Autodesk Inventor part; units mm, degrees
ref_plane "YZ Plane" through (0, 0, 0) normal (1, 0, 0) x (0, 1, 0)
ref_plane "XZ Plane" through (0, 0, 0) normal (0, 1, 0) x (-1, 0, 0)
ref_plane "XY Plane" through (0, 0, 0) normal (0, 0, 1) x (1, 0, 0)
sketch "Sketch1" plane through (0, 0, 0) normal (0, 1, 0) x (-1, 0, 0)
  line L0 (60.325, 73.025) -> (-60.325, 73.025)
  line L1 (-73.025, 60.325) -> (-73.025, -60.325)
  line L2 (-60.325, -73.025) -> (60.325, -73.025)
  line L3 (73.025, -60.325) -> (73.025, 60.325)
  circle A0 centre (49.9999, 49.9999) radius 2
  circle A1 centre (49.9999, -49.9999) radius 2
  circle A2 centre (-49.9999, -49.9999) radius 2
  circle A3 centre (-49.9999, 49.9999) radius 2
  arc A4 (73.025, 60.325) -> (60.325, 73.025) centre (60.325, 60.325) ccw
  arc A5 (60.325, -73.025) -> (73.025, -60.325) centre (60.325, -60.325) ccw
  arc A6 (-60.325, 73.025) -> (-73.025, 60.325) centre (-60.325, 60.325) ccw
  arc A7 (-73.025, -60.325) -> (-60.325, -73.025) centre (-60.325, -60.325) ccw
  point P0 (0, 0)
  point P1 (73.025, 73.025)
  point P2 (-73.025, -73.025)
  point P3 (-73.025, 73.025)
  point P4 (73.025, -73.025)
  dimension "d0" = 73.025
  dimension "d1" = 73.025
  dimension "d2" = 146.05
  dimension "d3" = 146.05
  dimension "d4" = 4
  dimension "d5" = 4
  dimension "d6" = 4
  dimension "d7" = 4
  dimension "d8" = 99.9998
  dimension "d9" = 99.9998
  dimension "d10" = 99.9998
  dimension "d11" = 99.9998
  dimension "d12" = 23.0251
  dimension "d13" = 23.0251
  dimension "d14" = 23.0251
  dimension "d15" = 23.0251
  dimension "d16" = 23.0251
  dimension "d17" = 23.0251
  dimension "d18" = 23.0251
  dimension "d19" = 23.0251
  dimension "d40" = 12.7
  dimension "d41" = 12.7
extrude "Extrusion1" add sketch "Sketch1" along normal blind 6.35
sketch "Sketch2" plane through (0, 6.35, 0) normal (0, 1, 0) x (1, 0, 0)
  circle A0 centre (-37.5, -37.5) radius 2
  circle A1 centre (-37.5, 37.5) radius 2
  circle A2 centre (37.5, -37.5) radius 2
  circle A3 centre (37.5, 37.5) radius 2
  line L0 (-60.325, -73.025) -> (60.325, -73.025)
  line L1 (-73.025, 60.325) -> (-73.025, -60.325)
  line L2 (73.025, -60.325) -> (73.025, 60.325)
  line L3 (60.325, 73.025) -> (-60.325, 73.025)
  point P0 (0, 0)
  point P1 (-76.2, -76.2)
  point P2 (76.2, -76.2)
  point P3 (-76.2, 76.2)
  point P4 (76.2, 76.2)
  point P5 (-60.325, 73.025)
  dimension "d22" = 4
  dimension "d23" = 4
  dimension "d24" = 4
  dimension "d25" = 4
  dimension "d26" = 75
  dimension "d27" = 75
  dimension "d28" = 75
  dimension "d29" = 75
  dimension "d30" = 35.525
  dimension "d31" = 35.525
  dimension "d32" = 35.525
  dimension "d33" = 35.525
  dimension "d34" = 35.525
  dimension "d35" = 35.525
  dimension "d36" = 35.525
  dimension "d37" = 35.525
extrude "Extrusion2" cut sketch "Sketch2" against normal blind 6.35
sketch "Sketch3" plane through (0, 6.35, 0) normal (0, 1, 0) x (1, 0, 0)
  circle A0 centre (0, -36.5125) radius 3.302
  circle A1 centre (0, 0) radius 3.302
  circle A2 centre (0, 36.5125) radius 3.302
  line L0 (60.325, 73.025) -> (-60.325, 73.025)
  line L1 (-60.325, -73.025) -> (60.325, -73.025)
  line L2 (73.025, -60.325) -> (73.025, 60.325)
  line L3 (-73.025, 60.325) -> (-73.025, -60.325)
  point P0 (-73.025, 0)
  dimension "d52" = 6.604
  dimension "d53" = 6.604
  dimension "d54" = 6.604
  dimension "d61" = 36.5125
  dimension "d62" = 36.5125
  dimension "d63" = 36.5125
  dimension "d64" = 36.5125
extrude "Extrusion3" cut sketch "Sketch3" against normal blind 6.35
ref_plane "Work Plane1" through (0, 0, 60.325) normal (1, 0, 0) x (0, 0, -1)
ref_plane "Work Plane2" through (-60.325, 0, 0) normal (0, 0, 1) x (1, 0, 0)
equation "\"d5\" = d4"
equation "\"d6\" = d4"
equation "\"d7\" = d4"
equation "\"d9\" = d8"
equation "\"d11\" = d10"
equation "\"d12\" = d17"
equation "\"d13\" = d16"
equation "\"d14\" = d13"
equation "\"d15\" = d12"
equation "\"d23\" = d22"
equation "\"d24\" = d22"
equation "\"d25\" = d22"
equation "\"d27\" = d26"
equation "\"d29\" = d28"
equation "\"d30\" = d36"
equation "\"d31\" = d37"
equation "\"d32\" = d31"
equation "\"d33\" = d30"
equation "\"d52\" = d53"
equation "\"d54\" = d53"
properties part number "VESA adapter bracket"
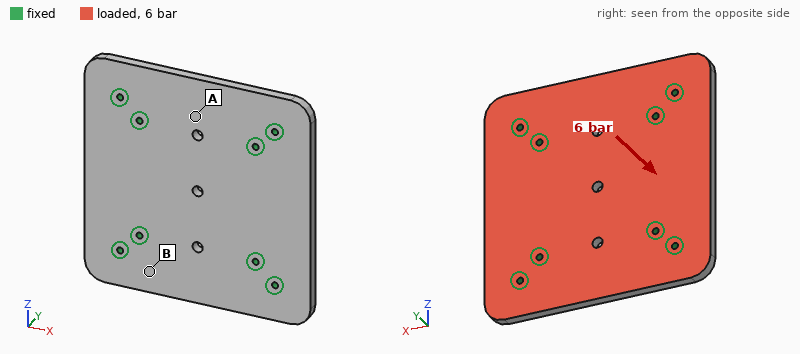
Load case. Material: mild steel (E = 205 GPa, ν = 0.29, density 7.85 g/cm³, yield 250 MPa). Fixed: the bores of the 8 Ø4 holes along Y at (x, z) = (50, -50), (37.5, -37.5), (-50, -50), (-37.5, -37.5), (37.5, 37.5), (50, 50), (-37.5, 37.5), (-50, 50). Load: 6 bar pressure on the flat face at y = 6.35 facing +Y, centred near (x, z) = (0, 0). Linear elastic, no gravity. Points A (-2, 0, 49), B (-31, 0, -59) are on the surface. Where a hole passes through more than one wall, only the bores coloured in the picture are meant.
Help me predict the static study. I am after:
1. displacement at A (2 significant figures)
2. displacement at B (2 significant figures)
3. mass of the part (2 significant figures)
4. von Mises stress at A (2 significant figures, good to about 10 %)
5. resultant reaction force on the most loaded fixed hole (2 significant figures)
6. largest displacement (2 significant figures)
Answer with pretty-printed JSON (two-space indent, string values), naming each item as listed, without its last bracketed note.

{
  "displacement at A": "21 µm",
  "displacement at B": "10 µm",
  "mass of the part": "1.0 kg",
  "von Mises stress at A": "30 MPa",
  "resultant reaction force on the most loaded fixed hole": "2.2 kN",
  "largest displacement": "31 µm"
}
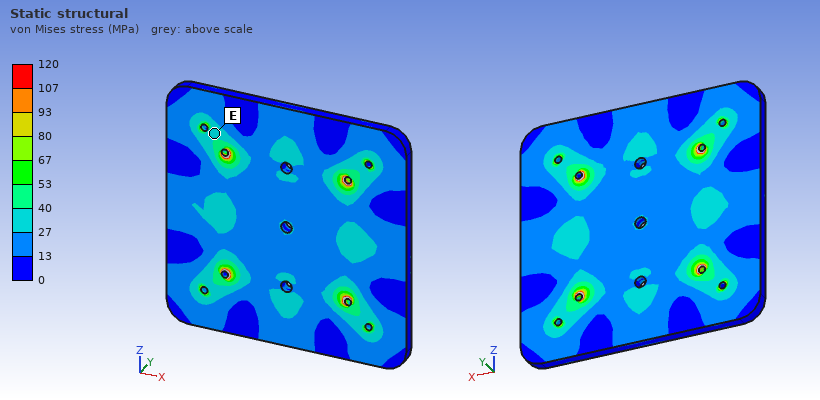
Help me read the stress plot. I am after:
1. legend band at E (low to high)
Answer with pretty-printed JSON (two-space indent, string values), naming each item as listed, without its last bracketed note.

{
  "legend band at E": "27 to 40 MPa"
}
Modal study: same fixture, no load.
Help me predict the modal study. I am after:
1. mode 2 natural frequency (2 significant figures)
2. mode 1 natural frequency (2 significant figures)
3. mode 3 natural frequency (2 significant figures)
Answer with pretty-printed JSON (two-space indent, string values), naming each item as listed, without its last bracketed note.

{
  "mode 2 natural frequency": "3700 Hz",
  "mode 1 natural frequency": "3400 Hz",
  "mode 3 natural frequency": "3700 Hz"
}
